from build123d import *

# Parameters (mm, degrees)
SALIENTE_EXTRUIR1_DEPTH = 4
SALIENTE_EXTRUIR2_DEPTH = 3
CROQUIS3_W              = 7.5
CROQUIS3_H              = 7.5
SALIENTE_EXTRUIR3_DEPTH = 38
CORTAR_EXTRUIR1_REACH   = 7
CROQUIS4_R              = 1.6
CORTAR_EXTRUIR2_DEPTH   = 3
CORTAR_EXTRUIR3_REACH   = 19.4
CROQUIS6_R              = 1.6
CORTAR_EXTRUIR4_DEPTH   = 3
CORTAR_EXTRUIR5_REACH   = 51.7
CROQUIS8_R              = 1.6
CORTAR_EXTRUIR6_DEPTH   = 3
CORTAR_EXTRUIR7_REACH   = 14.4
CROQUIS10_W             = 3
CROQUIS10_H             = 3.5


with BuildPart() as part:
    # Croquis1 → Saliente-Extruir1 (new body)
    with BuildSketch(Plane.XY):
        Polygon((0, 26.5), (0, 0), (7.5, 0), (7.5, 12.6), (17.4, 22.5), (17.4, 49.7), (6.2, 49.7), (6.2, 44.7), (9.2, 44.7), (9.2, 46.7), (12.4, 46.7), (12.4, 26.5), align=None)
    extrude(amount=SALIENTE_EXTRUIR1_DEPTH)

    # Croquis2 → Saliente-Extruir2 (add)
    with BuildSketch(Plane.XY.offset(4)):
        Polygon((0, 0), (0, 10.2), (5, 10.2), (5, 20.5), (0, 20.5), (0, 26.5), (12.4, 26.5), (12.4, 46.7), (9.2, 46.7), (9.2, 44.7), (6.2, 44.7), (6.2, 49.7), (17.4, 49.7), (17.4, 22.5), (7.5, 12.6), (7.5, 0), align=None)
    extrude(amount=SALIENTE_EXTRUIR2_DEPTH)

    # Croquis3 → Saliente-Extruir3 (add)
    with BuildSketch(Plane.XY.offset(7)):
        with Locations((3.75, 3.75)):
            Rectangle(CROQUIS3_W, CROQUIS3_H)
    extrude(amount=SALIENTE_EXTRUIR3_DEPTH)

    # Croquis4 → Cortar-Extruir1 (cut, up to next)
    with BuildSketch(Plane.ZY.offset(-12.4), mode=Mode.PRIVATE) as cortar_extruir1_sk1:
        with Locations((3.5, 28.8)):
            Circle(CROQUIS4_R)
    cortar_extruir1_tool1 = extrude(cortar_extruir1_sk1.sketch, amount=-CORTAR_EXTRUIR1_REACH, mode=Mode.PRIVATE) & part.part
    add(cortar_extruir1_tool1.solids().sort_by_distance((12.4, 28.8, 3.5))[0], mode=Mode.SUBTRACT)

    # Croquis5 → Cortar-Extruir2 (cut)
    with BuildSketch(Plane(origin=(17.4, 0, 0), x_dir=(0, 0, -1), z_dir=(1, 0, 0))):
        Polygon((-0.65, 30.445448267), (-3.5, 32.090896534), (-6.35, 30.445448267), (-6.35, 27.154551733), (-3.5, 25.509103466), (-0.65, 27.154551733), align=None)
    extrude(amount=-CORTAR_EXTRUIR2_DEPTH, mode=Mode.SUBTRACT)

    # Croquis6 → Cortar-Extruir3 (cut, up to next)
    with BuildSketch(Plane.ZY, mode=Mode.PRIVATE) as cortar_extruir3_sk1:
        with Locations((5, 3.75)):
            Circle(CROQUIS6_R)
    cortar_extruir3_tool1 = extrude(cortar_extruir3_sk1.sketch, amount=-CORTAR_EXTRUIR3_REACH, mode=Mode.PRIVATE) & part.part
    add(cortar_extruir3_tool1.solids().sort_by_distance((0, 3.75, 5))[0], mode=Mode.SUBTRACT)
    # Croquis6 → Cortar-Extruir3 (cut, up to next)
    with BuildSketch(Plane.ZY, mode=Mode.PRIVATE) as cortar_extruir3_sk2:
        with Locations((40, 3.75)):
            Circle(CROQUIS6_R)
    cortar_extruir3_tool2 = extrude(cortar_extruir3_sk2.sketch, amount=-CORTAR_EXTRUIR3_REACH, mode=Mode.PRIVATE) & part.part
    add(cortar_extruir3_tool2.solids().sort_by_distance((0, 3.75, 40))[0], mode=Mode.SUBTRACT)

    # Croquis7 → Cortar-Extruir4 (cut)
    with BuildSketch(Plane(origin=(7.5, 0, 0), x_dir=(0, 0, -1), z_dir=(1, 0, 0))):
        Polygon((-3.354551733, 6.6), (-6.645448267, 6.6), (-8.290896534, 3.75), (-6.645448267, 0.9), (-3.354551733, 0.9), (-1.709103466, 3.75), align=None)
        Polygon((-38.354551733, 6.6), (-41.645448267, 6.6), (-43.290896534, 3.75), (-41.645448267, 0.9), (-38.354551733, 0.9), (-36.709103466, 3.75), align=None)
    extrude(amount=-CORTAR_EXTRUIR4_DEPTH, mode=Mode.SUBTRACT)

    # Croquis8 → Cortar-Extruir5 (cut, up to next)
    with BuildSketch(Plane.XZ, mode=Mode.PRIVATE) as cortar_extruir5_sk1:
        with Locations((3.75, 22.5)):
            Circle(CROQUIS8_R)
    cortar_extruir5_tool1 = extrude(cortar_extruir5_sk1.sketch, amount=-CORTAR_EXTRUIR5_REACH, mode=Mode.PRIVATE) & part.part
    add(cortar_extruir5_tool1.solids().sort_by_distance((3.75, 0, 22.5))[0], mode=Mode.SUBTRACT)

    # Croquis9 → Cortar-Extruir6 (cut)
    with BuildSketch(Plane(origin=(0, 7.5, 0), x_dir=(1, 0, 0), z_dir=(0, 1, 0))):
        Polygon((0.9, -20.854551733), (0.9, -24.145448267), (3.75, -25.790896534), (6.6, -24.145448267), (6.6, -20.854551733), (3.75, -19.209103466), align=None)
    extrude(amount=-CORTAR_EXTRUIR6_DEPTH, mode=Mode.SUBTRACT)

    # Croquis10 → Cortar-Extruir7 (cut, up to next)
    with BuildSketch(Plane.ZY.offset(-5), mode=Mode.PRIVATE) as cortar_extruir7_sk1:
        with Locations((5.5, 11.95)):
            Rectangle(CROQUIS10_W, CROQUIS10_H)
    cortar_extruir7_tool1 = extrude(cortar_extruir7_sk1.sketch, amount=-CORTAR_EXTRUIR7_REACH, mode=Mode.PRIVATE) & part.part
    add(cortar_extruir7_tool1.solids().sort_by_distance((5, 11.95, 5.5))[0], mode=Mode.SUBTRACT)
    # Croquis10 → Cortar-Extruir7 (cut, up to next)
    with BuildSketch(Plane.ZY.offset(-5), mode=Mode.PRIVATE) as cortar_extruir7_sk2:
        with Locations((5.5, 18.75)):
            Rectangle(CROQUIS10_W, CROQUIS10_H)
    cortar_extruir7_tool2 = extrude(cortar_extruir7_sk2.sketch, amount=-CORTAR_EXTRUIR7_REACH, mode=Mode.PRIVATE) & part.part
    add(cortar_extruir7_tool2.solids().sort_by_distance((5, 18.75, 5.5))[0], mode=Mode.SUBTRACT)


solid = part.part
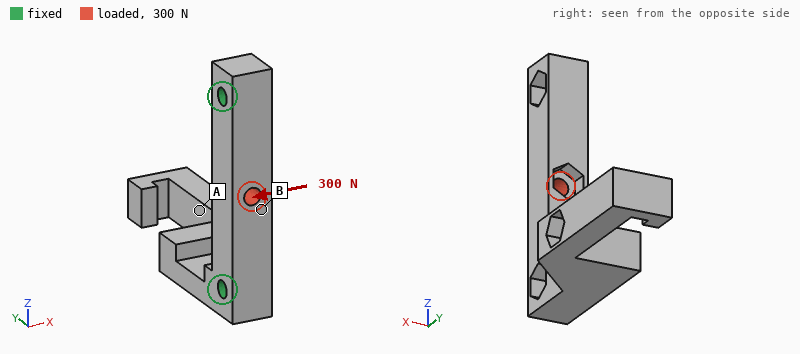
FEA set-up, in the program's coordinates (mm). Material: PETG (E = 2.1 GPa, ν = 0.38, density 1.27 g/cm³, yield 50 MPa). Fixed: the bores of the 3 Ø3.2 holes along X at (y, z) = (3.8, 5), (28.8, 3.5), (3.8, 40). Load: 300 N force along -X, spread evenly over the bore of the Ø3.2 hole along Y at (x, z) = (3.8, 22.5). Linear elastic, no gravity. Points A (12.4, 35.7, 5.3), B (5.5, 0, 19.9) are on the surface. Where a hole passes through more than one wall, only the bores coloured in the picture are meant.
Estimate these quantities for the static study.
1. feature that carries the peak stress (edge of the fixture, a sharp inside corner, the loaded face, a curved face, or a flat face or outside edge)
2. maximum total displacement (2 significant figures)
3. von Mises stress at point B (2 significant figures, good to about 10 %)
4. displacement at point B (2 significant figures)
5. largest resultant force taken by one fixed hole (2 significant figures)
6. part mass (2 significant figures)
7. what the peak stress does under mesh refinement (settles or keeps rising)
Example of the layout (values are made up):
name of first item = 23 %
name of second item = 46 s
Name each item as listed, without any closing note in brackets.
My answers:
feature that carries the peak stress = edge of the fixture
maximum total displacement = 0.30 mm
von Mises stress at point B = 15 MPa
displacement at point B = 0.27 mm
largest resultant force taken by one fixed hole = 190 N
part mass = 5.6 g
what the peak stress does under mesh refinement = keeps rising
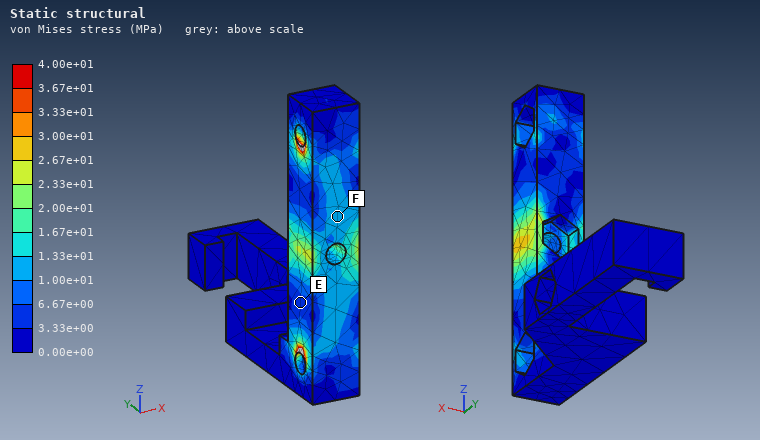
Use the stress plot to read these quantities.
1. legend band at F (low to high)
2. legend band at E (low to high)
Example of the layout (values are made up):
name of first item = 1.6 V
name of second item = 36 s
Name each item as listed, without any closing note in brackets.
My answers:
legend band at F = 1.00e+01 to 1.33e+01 MPa
legend band at E = 3.33e+00 to 6.67e+00 MPa
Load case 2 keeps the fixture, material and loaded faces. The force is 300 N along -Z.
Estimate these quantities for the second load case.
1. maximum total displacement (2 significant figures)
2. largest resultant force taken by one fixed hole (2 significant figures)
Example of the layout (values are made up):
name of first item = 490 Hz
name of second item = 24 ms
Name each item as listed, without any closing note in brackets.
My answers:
maximum total displacement = 35 µm
largest resultant force taken by one fixed hole = 150 N
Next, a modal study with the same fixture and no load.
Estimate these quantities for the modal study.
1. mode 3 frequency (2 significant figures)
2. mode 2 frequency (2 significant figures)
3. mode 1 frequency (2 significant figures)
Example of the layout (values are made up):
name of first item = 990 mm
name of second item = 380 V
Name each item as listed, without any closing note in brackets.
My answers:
mode 3 frequency = 3700 Hz
mode 2 frequency = 1700 Hz
mode 1 frequency = 1200 Hz
